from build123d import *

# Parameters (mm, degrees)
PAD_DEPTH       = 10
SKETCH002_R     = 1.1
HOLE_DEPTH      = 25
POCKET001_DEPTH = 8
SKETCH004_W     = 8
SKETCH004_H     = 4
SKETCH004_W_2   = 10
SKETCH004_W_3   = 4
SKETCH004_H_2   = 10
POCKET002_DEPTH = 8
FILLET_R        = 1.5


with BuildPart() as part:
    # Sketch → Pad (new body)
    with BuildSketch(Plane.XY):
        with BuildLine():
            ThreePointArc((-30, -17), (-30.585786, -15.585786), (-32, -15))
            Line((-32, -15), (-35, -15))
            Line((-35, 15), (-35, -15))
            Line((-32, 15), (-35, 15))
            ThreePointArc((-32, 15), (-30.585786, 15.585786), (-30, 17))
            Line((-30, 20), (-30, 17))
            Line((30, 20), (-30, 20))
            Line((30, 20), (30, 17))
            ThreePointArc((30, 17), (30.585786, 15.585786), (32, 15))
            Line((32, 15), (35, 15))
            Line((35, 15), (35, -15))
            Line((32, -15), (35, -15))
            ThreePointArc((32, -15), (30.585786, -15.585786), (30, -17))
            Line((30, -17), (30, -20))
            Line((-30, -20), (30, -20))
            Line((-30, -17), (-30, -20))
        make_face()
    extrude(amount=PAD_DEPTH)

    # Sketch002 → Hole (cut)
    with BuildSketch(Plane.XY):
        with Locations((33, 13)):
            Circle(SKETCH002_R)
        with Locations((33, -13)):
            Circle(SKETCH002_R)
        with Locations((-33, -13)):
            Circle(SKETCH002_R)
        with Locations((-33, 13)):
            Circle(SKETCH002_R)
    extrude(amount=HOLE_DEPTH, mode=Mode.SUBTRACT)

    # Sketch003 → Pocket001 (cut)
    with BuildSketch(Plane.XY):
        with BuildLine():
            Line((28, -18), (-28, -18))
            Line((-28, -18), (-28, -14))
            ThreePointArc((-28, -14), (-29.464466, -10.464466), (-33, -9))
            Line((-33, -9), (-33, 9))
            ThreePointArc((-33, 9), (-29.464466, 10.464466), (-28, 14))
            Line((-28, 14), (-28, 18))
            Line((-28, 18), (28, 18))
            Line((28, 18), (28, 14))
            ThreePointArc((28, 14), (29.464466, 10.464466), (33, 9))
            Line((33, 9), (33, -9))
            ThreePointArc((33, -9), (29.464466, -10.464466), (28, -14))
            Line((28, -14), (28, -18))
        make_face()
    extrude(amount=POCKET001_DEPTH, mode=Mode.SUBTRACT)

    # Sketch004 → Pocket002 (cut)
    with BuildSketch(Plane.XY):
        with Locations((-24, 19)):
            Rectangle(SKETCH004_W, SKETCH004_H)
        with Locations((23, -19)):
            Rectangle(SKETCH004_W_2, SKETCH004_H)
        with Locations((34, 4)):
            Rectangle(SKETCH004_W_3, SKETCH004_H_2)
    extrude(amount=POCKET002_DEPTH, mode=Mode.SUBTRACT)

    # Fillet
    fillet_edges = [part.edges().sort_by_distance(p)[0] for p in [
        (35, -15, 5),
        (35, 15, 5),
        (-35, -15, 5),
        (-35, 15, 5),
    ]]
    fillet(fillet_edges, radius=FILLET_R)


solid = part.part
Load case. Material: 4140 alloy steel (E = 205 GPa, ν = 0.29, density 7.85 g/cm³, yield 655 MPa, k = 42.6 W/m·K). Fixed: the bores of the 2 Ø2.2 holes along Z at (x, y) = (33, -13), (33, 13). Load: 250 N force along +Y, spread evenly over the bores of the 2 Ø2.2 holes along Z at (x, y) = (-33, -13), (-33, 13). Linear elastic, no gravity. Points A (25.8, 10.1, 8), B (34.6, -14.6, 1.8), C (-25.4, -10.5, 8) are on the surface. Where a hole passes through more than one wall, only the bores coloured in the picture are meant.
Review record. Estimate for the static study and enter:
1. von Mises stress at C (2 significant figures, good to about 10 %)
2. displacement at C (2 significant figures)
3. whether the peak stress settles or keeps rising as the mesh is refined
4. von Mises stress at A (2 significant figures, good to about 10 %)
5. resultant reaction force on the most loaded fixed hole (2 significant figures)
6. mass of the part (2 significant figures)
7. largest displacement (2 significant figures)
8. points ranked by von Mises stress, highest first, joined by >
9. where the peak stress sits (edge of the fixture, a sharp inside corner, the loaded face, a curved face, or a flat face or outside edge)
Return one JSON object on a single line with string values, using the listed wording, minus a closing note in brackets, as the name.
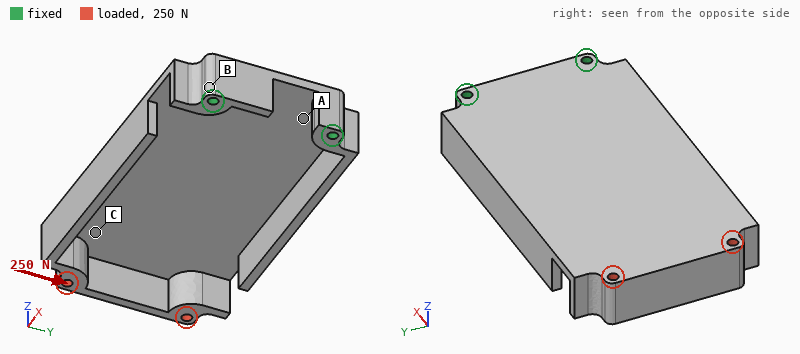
{"von Mises stress at C": "23 MPa", "displacement at C": "0.066 mm", "whether the peak stress settles or keeps rising as the mesh is refined": "keeps rising", "von Mises stress at A": "32 MPa", "resultant reaction force on the most loaded fixed hole": "630 N", "mass of the part": "68 g", "largest displacement": "0.12 mm", "points ranked by von Mises stress, highest first, joined by >": "A > C > B", "where the peak stress sits": "edge of the fixture"}
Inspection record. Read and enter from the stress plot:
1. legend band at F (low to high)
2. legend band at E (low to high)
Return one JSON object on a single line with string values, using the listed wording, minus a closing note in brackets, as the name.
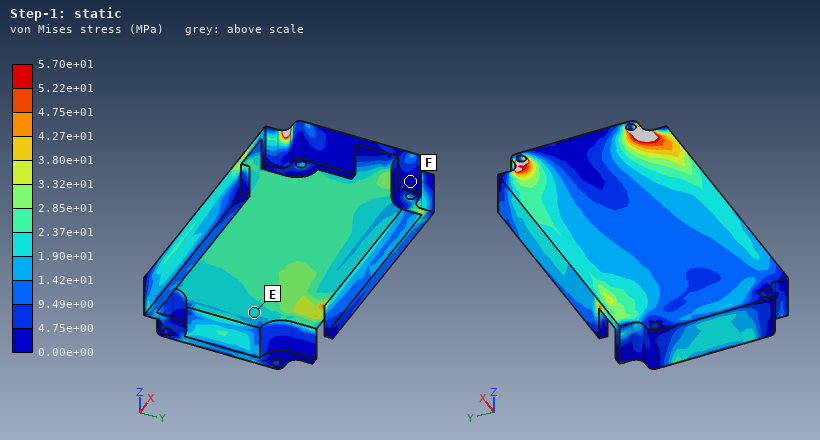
{"legend band at F": "0.00e+00 to 4.75e+00 MPa", "legend band at E": "1.90e+01 to 2.37e+01 MPa"}
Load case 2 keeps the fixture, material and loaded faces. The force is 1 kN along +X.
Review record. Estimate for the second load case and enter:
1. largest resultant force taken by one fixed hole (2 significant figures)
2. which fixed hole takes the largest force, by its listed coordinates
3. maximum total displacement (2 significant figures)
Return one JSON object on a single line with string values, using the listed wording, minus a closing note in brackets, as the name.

{"largest resultant force taken by one fixed hole": "540 N", "which fixed hole takes the largest force, by its listed coordinates": "(33, -13)", "maximum total displacement": "0.42 mm"}
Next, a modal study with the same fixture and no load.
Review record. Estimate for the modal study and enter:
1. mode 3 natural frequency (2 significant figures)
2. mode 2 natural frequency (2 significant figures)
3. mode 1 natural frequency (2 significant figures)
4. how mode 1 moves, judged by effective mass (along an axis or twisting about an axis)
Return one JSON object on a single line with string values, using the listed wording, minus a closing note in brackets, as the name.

{"mode 3 natural frequency": "4100 Hz", "mode 2 natural frequency": "1600 Hz", "mode 1 natural frequency": "550 Hz", "how mode 1 moves, judged by effective mass": "along Z"}
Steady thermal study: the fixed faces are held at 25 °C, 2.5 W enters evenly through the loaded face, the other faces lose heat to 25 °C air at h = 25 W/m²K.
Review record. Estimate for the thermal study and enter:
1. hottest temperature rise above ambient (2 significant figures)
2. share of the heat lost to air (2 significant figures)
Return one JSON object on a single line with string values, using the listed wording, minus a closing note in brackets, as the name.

{"hottest temperature rise above ambient": "21 K", "share of the heat lost to air": "70 %"}
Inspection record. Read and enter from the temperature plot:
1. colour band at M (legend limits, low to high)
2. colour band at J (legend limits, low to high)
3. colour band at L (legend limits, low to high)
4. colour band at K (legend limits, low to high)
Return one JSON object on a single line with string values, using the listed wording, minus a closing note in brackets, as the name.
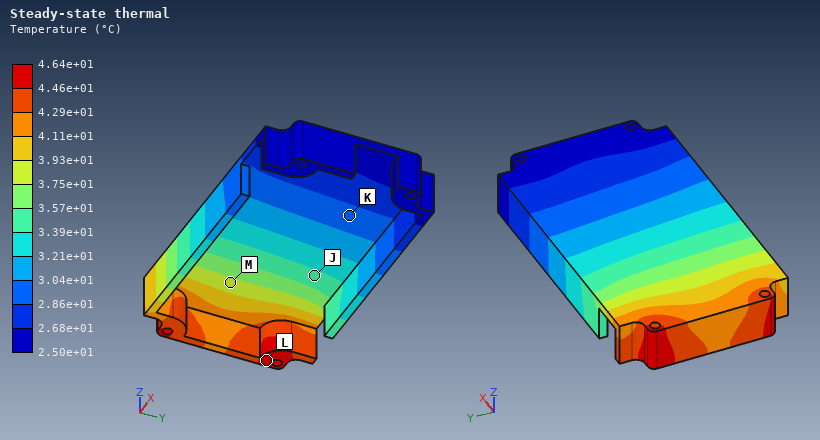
{"colour band at M": "3.75e+01 to 3.93e+01 °C", "colour band at J": "3.39e+01 to 3.57e+01 °C", "colour band at L": "4.46e+01 to 4.64e+01 °C", "colour band at K": "2.86e+01 to 3.04e+01 °C"}
